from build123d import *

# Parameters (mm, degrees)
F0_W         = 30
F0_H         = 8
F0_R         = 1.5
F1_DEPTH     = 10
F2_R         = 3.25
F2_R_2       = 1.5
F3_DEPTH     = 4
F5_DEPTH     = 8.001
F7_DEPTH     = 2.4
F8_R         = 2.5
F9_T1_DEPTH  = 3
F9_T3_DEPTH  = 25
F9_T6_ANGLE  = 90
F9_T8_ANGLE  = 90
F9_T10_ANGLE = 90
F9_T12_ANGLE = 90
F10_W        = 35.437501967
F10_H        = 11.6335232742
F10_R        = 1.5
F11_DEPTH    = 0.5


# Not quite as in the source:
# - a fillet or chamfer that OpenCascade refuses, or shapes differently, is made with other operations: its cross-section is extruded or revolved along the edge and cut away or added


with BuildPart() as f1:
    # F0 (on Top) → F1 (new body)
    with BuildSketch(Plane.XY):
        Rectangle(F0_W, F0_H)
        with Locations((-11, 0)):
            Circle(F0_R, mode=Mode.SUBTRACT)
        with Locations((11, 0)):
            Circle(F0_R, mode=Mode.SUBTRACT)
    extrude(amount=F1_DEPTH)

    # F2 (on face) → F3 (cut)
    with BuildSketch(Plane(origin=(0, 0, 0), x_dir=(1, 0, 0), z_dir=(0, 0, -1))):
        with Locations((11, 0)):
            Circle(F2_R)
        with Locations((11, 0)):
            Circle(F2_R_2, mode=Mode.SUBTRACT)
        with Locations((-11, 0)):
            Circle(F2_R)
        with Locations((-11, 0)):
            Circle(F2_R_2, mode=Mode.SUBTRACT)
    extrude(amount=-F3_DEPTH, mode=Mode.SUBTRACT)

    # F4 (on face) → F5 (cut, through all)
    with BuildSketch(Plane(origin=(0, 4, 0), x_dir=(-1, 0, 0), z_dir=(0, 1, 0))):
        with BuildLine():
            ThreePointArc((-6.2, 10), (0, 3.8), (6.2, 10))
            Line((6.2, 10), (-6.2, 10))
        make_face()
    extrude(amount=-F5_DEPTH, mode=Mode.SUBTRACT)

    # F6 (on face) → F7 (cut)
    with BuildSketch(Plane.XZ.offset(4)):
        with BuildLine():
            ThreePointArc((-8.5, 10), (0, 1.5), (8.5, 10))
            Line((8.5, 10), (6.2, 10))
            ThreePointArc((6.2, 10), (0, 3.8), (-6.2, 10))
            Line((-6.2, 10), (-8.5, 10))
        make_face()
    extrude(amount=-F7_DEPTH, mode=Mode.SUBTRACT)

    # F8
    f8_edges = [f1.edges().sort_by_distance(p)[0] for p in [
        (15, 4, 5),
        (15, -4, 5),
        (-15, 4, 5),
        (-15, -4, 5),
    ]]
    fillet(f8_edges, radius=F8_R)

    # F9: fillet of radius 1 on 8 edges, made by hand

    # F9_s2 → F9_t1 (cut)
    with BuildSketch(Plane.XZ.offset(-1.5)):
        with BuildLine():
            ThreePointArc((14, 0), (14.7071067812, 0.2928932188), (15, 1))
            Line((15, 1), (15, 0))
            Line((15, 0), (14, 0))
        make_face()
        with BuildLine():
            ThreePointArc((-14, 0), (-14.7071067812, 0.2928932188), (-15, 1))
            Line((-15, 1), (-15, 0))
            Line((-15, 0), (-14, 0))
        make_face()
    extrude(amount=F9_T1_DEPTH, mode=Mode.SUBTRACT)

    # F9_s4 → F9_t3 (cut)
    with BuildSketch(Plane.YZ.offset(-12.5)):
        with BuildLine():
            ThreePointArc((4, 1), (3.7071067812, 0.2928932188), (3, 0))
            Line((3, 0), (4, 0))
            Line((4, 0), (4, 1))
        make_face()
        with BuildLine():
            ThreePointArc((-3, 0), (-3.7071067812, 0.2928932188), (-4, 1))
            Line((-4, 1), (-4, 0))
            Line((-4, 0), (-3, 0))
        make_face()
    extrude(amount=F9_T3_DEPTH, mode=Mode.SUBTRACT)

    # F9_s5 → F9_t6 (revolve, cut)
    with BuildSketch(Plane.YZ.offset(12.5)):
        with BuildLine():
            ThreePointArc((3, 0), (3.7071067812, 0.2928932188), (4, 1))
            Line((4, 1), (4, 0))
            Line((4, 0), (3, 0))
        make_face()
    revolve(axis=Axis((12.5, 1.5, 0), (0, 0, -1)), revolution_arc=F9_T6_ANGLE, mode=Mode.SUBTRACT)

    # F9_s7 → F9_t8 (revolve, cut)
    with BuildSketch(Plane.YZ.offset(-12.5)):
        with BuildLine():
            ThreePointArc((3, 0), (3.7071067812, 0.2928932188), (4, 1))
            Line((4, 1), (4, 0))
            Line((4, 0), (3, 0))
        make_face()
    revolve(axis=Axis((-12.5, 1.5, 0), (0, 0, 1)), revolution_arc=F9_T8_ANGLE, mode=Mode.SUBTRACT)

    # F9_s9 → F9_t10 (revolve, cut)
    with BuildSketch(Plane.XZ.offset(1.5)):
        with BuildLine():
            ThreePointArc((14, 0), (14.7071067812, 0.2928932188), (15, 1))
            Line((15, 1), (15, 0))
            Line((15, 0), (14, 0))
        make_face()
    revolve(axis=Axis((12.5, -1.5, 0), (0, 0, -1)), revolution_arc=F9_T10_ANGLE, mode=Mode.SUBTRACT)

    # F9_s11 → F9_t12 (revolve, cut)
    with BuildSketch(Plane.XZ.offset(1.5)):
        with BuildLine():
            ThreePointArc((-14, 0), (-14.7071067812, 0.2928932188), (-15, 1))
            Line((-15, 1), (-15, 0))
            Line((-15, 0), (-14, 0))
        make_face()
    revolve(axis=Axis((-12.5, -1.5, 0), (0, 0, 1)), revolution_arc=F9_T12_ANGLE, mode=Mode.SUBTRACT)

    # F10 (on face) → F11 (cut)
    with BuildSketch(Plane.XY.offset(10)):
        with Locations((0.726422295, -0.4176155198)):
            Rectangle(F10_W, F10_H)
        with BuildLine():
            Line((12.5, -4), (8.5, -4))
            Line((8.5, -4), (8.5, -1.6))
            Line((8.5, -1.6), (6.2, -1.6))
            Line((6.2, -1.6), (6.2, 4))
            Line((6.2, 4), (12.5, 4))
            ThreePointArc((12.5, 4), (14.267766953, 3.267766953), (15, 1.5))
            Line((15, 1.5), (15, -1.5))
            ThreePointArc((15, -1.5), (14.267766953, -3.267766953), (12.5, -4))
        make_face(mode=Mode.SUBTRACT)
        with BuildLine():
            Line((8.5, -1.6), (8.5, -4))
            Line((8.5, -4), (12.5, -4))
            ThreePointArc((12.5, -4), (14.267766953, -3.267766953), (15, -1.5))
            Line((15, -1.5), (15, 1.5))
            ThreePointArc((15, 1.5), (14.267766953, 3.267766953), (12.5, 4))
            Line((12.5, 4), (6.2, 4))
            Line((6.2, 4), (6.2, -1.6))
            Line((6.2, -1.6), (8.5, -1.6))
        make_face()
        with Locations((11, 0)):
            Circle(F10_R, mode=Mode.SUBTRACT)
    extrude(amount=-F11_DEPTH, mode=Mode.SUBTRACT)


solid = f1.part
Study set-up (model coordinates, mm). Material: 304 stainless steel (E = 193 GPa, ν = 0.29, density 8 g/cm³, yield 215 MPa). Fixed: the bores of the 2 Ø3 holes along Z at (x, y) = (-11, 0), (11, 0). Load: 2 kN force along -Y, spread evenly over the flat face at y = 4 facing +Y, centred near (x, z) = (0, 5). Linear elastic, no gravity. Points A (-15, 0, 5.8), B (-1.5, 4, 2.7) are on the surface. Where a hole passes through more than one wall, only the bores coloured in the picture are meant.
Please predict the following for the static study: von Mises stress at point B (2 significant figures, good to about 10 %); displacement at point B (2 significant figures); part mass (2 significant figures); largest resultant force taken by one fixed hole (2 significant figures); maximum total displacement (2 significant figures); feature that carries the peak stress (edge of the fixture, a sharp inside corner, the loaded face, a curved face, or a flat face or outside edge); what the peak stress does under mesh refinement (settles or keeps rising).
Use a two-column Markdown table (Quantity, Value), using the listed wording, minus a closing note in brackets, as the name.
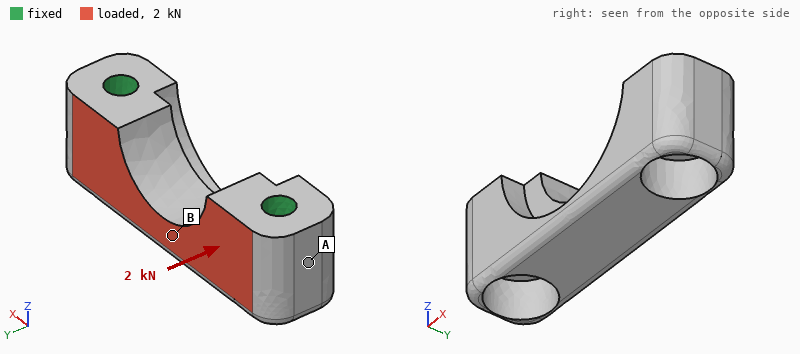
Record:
| Quantity | Value |
|---|---|
| von Mises stress at point B | 28 MPa |
| displacement at point B | 4.3 µm |
| part mass | 11 g |
| largest resultant force taken by one fixed hole | 1.0 kN |
| maximum total displacement | 5.1 µm |
| feature that carries the peak stress | edge of the fixture |
| what the peak stress does under mesh refinement | keeps rising |
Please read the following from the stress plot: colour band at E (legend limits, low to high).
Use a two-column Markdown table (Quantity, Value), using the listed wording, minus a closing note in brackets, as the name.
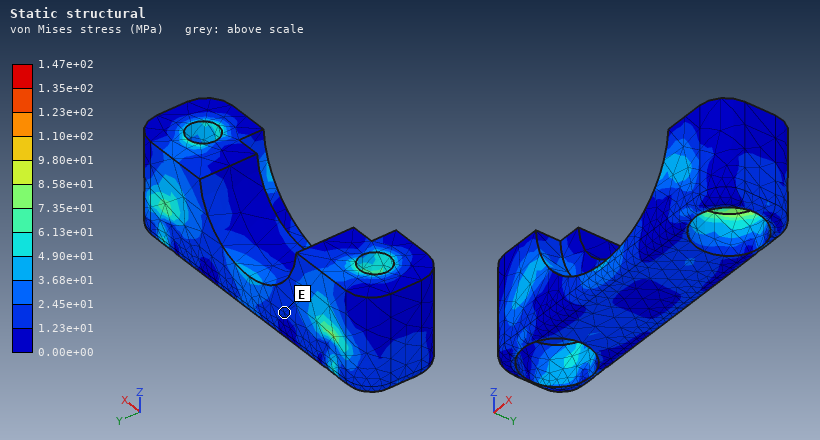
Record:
| Quantity | Value |
|---|---|
| colour band at E | 1.23e+01 to 2.45e+01 MPa |
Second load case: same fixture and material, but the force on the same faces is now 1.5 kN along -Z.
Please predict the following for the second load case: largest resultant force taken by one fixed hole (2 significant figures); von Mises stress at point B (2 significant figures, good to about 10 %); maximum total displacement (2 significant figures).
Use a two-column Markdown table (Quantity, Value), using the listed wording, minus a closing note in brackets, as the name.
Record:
| Quantity | Value |
|---|---|
| largest resultant force taken by one fixed hole | 780 N |
| von Mises stress at point B | 28 MPa |
| maximum total displacement | 4.5 µm |
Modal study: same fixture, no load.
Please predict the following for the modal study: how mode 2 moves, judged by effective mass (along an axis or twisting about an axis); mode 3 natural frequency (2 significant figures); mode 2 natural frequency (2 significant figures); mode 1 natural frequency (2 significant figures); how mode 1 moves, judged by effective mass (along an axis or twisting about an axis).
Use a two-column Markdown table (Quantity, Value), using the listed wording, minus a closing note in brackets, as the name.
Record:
| Quantity | Value |
|---|---|
| how mode 2 moves, judged by effective mass | along Z |
| mode 3 natural frequency | 61 kHz |
| mode 2 natural frequency | 59 kHz |
| mode 1 natural frequency | 36 kHz |
| how mode 1 moves, judged by effective mass | along Y |
